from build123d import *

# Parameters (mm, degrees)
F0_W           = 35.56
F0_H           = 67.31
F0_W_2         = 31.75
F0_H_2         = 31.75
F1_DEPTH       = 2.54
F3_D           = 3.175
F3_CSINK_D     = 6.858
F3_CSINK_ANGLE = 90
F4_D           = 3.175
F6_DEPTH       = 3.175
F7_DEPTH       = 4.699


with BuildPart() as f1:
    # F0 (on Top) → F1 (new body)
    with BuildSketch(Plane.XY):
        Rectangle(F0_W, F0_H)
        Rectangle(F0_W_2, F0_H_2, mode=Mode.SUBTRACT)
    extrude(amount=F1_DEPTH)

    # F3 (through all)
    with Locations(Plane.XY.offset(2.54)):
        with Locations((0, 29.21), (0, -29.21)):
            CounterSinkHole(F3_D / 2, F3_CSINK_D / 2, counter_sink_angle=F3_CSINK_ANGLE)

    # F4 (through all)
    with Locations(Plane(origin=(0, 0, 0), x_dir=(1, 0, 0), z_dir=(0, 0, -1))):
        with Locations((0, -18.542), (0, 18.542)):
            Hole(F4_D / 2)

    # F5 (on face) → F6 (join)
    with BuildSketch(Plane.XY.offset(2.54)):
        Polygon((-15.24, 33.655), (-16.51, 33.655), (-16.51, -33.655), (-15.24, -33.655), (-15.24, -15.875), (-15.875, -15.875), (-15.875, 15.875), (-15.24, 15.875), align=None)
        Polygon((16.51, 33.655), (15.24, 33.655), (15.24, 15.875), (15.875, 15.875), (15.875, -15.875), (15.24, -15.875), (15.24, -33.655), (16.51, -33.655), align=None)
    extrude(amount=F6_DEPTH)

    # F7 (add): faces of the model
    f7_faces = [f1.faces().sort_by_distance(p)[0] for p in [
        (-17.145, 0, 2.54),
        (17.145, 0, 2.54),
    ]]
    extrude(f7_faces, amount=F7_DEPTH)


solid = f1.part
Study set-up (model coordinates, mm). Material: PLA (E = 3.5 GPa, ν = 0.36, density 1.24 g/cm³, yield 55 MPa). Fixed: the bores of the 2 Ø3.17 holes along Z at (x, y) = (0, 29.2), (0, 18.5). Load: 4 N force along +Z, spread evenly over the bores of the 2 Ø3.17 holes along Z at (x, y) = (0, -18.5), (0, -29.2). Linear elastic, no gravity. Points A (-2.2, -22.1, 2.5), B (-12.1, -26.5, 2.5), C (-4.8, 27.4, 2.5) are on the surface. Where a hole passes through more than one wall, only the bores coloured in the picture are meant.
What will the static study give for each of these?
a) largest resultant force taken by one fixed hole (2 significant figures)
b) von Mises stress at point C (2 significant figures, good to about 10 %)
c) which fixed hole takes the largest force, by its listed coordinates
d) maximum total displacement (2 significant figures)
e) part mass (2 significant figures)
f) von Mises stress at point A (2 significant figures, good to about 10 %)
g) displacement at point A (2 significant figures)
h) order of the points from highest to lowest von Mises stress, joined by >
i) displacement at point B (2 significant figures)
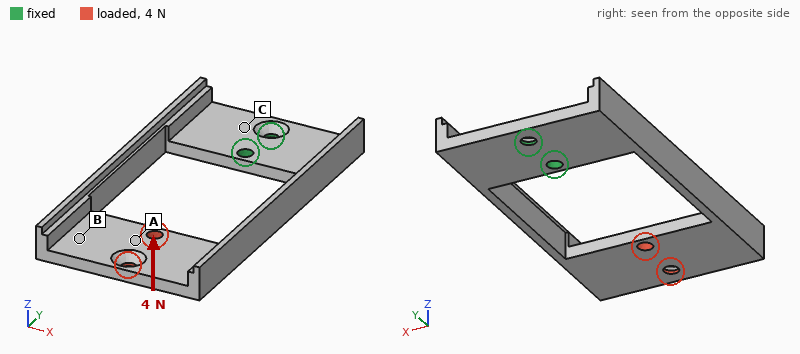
18 N
2.7 MPa
(0, 18.5)
0.91 mm
5.7 g
2.0 MPa
0.71 mm
C > A > B
0.76 mm
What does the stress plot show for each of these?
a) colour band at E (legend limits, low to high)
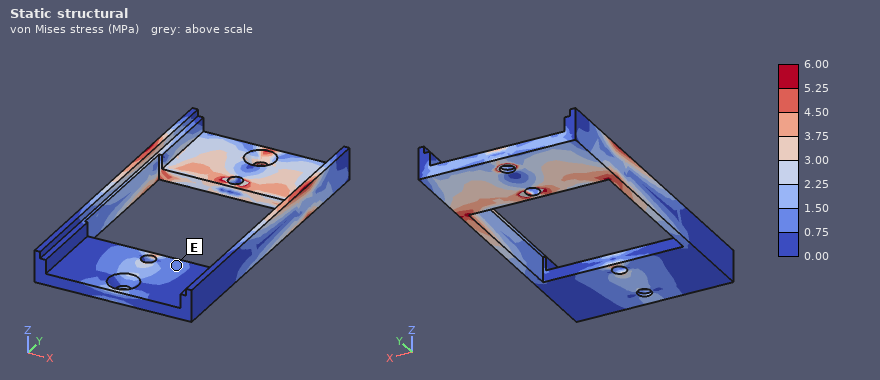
0.75 to 1.50 MPa
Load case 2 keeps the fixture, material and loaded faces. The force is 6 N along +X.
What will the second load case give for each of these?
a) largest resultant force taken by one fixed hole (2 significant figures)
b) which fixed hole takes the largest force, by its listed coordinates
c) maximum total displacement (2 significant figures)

25 N
(0, 18.5)
0.85 mm
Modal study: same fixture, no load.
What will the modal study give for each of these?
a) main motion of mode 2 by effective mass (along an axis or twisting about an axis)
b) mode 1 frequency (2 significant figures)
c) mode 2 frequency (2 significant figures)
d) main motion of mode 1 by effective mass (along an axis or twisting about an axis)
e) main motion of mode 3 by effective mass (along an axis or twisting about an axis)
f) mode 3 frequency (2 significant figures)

along X
220 Hz
260 Hz
along Z
twisting about Y
450 Hz
